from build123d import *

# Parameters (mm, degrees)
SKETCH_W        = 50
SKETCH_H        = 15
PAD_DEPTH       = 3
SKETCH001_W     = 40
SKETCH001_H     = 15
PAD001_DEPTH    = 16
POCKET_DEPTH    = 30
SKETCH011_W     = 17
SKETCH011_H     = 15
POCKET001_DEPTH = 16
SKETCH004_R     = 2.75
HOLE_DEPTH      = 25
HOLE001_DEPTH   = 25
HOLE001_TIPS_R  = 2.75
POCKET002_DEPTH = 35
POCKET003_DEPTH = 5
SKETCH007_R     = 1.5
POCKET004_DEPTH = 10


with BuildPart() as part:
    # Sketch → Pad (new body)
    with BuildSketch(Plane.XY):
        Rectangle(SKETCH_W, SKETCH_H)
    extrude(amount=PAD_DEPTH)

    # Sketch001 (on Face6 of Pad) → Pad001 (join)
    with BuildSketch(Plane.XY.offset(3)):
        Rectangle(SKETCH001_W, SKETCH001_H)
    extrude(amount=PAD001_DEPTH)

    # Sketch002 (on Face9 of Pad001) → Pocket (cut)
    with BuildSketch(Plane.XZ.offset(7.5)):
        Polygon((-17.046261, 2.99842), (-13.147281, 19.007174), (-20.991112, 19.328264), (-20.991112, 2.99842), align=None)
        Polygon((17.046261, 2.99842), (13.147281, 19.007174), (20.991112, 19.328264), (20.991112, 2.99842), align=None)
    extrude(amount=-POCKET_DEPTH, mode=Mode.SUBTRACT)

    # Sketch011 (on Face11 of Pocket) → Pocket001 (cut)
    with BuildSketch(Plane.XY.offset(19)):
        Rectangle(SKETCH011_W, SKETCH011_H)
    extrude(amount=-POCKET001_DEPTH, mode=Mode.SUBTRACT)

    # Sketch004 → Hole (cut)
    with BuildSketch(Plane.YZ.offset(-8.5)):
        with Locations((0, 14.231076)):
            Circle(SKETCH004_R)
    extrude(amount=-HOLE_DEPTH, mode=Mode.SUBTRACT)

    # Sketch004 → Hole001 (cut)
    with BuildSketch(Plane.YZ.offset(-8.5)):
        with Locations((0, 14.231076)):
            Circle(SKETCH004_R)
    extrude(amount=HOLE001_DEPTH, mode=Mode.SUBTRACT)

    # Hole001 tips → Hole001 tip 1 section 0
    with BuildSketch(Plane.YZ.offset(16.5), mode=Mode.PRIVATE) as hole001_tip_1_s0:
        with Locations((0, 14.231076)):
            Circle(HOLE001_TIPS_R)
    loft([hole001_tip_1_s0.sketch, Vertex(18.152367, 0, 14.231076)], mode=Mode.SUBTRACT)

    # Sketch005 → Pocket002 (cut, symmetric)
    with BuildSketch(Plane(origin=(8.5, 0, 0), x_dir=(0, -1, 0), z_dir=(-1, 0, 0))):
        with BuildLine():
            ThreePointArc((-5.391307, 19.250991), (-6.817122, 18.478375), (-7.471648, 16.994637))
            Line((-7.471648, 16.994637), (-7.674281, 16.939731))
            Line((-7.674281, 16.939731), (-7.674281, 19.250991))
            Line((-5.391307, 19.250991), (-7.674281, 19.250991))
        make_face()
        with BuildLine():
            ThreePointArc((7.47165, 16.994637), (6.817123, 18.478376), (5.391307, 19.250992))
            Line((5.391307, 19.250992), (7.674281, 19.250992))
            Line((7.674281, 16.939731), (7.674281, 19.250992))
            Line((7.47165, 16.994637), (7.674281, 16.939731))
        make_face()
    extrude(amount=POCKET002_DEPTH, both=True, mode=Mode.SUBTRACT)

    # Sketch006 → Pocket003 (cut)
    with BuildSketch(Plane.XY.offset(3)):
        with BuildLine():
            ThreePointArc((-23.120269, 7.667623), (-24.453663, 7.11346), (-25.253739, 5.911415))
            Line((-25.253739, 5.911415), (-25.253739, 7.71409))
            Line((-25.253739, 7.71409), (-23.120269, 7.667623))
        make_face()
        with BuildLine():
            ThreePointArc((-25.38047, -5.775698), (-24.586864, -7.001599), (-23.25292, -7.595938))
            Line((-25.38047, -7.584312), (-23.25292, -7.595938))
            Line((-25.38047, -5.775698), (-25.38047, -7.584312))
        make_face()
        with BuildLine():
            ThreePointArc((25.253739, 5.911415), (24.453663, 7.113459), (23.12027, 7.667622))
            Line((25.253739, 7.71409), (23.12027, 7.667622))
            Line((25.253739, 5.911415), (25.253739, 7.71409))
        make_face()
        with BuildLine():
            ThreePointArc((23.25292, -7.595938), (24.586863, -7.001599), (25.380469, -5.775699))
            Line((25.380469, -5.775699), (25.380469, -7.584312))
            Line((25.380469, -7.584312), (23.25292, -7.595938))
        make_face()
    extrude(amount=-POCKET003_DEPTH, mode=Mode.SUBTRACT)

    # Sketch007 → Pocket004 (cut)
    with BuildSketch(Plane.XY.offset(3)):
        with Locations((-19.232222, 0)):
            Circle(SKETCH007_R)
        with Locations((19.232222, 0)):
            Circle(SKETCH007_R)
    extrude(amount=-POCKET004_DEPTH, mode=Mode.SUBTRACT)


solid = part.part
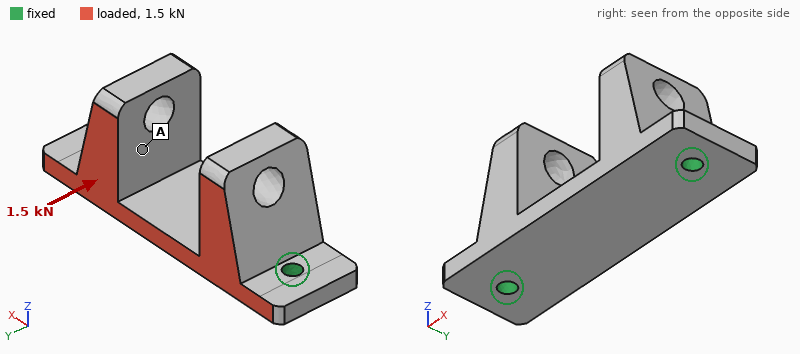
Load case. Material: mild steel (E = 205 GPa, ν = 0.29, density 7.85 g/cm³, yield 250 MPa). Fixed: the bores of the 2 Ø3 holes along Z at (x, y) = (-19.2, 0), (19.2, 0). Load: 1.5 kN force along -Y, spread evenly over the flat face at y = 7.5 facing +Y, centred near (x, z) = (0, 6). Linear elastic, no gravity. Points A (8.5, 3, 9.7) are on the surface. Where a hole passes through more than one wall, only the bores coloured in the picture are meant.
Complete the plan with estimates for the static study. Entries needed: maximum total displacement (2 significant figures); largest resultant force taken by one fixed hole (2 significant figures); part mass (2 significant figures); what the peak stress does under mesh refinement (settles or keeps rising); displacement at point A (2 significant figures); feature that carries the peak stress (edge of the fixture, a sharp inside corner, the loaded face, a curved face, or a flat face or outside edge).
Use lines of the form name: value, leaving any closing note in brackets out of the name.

maximum total displacement: 22 µm
largest resultant force taken by one fixed hole: 750 N
part mass: 40 g
what the peak stress does under mesh refinement: keeps rising
displacement at point A: 12 µm
feature that carries the peak stress: edge of the fixture
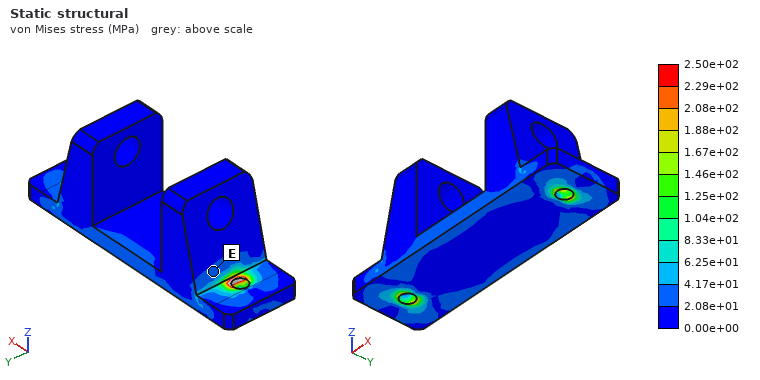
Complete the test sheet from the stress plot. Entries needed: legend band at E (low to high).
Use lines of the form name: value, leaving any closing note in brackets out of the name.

legend band at E: 2.08e+01 to 4.17e+01 MPa
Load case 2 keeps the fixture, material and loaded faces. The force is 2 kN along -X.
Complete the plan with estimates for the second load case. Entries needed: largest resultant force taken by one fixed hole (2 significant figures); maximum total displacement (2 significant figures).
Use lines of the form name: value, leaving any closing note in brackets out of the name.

largest resultant force taken by one fixed hole: 1.1 kN
maximum total displacement: 16 µm
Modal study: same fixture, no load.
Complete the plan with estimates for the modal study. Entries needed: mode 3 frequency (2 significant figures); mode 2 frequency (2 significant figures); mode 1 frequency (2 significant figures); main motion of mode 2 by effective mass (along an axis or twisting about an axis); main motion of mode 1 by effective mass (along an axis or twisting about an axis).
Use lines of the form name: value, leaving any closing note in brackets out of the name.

mode 3 frequency: 9300 Hz
mode 2 frequency: 7600 Hz
mode 1 frequency: 5700 Hz
main motion of mode 2 by effective mass: along Y
main motion of mode 1 by effective mass: along Z
